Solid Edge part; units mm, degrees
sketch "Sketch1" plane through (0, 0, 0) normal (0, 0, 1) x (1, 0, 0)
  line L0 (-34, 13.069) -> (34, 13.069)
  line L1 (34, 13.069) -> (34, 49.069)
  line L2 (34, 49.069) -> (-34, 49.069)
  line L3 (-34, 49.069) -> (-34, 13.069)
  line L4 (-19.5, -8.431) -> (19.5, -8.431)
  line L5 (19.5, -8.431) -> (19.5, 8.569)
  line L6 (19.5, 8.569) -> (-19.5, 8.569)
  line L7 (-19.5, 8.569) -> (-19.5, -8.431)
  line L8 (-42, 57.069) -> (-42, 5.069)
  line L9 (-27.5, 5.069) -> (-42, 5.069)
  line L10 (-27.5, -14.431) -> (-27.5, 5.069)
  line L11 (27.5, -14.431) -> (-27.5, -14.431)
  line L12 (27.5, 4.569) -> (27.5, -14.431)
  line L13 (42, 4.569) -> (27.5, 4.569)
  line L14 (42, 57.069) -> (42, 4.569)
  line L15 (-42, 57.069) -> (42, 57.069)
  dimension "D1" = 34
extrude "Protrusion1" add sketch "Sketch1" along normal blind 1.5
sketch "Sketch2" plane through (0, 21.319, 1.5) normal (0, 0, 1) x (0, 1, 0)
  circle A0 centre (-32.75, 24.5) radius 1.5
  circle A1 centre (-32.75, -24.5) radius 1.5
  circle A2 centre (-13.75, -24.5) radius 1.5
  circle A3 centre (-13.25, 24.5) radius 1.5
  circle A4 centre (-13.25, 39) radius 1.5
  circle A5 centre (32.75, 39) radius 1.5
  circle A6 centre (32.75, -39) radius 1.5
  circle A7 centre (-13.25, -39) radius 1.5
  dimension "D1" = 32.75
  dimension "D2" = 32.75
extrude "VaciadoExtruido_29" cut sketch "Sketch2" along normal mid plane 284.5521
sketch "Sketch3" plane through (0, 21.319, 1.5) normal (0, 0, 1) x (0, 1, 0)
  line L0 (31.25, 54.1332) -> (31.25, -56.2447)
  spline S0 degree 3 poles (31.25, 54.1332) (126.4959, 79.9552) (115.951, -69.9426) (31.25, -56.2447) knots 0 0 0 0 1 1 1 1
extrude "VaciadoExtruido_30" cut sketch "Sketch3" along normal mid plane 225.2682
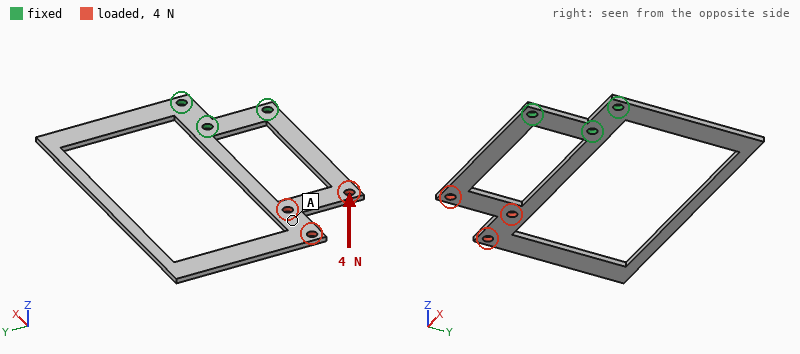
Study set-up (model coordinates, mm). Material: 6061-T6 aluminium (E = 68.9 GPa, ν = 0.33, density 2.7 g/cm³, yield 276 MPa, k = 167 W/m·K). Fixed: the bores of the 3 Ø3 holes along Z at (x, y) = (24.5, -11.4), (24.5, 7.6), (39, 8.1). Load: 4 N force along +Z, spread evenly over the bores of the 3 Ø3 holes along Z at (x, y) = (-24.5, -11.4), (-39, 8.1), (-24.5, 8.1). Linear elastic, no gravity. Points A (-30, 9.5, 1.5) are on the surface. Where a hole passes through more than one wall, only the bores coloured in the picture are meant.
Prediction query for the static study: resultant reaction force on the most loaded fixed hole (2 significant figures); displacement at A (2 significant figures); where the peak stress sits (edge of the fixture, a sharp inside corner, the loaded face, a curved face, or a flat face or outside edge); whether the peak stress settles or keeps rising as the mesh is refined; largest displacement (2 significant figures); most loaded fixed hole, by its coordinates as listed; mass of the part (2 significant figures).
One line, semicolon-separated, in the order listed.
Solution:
2.8 N; 0.84 mm; a sharp inside corner; keeps rising; 1.1 mm; (24.5, 7.6); 7.8 g
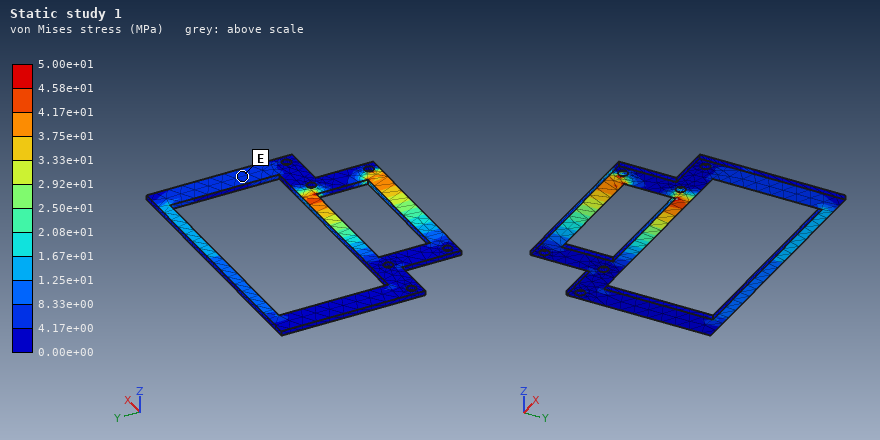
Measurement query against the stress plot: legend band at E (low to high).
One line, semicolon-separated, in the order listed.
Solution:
4.17e+00 to 8.33e+00 MPa
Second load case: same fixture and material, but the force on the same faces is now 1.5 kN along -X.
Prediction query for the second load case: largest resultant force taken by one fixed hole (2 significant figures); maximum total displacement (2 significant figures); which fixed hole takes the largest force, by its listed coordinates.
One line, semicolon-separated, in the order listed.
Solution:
770 N; 0.12 mm; (24.5, 7.6)
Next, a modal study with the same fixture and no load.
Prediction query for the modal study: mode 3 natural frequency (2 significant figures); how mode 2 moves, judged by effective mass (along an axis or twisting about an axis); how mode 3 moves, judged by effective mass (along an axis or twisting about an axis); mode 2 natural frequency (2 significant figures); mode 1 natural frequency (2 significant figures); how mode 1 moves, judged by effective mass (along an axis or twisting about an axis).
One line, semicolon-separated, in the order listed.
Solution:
620 Hz; twisting about X; along Z; 390 Hz; 160 Hz; along Z
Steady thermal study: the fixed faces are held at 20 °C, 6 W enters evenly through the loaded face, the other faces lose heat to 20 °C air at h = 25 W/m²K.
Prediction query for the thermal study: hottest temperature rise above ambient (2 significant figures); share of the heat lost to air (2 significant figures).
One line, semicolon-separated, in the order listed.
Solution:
62 K; 49 %
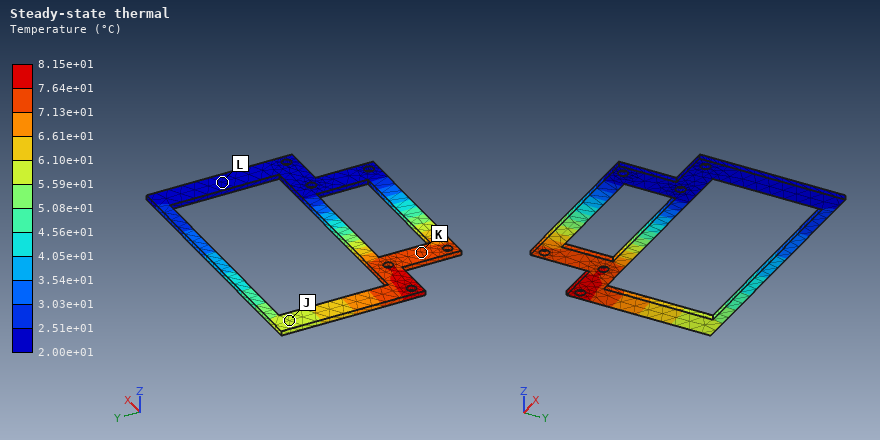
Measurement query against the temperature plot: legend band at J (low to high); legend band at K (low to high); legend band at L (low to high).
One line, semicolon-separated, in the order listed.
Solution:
5.59e+01 to 6.10e+01 °C; 7.13e+01 to 7.64e+01 °C; 2.00e+01 to 2.51e+01 °C
